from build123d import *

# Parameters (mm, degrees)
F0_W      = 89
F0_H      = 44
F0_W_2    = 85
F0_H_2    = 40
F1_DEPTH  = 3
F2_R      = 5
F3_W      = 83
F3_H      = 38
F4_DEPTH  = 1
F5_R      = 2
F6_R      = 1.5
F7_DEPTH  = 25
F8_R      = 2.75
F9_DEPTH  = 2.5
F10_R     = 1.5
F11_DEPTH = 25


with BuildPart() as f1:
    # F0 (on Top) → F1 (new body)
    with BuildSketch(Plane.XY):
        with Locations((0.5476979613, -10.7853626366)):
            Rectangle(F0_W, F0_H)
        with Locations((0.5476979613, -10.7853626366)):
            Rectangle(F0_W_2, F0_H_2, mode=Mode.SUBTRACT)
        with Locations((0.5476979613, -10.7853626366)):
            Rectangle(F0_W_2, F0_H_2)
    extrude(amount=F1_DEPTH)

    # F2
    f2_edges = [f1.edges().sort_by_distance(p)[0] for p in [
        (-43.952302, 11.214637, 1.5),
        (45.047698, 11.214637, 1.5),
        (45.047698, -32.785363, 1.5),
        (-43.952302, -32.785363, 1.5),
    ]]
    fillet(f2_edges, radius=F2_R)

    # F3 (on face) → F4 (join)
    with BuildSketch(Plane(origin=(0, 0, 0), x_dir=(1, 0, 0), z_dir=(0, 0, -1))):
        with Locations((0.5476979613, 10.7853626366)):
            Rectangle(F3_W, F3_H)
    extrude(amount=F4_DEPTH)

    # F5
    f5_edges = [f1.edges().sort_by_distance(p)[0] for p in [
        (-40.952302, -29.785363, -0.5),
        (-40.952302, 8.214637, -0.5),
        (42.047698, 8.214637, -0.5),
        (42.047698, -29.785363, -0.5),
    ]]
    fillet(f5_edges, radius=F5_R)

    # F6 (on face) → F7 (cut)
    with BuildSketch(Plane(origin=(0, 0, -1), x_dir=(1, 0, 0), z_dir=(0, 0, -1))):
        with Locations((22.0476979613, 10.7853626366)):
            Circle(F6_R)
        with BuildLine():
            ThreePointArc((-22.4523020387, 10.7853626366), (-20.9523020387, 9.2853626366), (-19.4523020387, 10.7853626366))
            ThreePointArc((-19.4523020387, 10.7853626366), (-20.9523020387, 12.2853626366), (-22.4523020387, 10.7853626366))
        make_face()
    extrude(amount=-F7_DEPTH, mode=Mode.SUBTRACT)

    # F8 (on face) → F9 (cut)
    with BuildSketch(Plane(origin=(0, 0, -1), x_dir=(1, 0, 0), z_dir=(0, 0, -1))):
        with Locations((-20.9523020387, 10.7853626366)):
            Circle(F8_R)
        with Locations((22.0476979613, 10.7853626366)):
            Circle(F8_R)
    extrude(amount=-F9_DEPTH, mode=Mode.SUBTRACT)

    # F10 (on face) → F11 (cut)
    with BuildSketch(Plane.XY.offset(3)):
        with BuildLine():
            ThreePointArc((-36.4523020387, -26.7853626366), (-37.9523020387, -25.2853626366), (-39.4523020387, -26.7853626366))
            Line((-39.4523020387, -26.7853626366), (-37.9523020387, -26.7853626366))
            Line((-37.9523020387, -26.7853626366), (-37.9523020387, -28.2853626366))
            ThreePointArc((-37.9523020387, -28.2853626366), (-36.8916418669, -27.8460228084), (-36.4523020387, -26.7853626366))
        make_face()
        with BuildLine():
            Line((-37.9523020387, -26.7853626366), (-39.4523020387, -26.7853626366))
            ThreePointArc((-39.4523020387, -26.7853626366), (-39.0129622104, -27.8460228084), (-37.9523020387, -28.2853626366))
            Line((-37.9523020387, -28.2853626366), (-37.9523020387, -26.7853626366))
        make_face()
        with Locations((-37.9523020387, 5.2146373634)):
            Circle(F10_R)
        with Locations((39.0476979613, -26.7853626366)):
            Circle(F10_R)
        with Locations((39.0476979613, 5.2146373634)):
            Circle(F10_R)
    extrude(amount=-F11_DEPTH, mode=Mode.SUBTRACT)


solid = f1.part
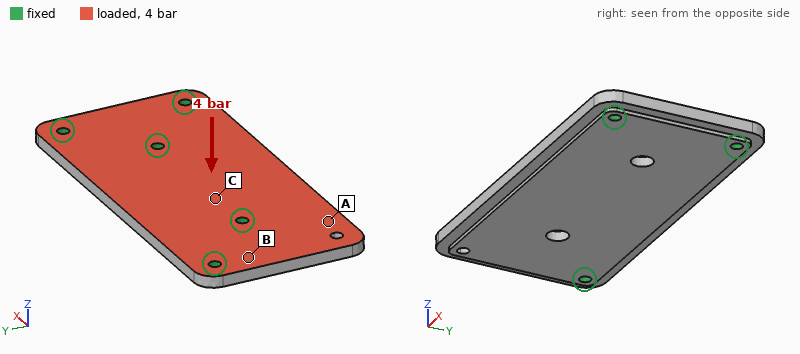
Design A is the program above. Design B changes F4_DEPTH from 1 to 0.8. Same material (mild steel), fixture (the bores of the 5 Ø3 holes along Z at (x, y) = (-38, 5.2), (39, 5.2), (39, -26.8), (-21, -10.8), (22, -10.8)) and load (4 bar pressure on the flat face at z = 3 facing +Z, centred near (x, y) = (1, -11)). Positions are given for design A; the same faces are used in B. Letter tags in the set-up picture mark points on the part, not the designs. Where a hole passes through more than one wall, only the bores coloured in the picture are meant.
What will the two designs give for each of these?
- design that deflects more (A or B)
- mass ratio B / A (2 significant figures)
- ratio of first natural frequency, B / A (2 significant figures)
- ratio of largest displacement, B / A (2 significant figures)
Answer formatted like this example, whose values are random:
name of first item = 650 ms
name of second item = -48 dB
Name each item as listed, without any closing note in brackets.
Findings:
design that deflects more = B
mass ratio B / A = 0.96
ratio of first natural frequency, B / A = 0.96
ratio of largest displacement, B / A = 1.1
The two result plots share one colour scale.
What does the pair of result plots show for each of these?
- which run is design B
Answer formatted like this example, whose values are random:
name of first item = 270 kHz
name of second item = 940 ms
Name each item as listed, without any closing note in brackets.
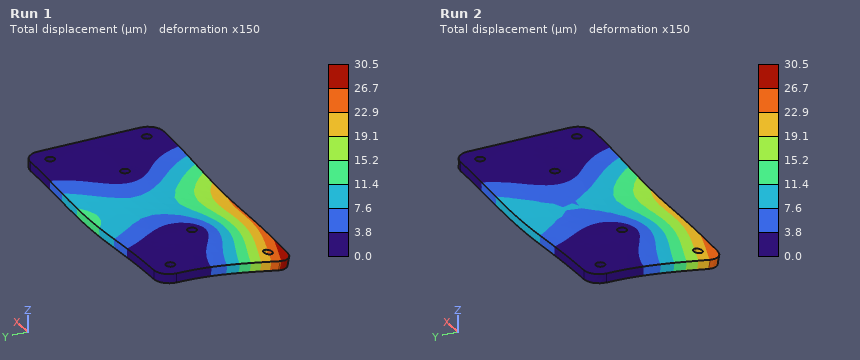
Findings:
which run is design B = Run 1
